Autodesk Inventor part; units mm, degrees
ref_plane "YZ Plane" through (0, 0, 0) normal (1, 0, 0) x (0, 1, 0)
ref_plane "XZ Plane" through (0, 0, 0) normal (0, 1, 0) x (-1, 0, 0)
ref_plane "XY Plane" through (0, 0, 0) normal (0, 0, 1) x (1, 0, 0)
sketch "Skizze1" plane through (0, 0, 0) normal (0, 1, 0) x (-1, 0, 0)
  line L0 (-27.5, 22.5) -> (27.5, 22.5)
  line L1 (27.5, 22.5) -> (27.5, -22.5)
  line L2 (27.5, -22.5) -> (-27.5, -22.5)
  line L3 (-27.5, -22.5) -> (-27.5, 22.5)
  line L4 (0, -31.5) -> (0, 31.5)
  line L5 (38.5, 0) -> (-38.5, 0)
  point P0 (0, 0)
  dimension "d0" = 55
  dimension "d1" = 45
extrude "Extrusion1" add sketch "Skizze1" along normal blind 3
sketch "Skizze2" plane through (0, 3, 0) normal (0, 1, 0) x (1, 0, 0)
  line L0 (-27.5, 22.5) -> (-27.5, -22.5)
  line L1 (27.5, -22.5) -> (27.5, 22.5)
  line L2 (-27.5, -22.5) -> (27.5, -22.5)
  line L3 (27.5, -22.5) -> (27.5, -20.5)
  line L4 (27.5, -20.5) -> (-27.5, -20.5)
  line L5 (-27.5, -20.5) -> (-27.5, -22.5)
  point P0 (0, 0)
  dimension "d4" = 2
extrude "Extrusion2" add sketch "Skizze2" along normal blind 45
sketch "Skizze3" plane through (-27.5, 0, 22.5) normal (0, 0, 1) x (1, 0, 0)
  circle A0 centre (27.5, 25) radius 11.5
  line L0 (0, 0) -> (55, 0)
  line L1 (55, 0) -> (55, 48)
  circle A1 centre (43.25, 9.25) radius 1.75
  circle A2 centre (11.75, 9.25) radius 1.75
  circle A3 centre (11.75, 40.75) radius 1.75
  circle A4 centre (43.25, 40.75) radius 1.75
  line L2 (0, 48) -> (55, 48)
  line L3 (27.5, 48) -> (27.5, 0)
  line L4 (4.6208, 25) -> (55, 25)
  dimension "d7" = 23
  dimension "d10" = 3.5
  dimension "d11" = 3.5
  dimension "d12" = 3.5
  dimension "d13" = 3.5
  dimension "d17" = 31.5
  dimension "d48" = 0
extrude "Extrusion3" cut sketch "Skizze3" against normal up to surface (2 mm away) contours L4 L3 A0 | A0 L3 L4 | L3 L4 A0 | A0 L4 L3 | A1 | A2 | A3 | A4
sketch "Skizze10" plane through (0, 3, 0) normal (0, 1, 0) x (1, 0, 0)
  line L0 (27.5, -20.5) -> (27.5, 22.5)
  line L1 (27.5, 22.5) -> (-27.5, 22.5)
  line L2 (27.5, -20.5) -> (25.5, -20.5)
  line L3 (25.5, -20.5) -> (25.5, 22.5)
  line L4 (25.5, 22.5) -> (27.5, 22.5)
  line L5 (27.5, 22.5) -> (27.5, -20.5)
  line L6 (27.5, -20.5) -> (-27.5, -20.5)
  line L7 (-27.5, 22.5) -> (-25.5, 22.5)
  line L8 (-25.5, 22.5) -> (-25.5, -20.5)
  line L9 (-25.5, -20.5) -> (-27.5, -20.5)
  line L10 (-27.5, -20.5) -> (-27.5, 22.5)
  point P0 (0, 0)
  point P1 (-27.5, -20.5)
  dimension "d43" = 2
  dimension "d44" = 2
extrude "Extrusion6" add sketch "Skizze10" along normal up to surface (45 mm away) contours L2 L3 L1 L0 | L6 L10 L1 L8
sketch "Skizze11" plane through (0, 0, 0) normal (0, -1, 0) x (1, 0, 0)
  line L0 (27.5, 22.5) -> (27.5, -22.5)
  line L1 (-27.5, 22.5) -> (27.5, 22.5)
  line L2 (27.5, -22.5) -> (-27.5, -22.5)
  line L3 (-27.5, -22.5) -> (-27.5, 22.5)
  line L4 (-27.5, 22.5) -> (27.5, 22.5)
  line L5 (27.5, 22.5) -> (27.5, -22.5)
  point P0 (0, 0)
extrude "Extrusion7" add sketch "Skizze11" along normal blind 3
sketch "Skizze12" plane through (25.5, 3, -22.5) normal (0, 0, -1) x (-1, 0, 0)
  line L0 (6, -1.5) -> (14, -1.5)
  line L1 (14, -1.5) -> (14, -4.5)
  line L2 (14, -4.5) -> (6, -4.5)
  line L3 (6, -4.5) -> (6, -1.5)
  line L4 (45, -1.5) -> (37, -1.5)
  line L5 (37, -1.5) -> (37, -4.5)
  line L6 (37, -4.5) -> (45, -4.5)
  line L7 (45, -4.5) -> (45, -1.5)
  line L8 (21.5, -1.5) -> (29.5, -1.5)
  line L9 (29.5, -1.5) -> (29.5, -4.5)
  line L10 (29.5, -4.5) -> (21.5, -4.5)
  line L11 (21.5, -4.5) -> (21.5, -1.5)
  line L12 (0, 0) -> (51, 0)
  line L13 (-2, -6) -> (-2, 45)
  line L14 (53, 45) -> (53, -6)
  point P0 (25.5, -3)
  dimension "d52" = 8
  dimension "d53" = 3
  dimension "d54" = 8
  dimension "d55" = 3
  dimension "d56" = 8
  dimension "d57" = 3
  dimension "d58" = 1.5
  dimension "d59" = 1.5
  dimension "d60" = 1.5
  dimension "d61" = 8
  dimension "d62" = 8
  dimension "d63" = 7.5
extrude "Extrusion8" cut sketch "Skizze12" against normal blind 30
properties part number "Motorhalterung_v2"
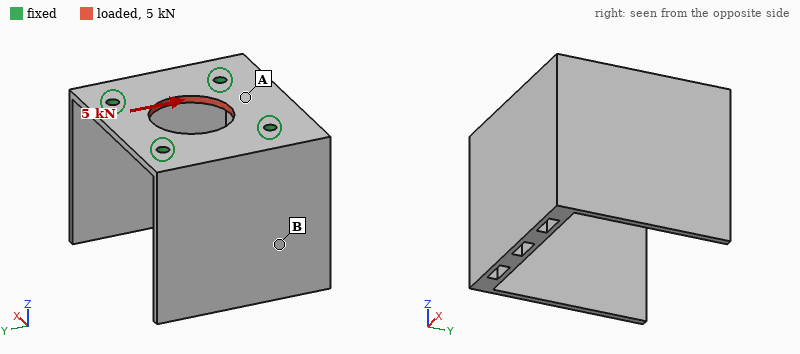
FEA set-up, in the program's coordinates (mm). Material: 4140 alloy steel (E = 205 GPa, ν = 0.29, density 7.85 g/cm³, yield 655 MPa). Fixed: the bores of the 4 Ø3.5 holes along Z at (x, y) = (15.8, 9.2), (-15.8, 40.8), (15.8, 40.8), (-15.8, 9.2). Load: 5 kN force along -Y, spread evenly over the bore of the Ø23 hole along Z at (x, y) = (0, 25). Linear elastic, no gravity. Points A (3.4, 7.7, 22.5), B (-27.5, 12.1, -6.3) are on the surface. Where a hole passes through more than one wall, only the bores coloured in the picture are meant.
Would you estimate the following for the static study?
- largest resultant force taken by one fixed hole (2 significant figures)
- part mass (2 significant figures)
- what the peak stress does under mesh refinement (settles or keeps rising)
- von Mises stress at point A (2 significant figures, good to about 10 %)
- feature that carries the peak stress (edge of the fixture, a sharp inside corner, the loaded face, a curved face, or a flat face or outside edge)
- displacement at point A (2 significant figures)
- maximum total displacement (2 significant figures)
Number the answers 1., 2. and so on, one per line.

1. 1.3 kN
2. 190 g
3. keeps rising
4. 25 MPa
5. edge of the fixture
6. 3.3 µm
7. 6.6 µm
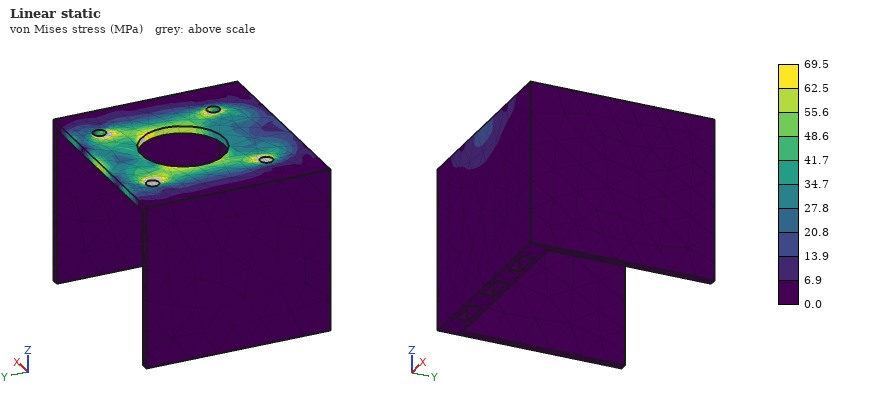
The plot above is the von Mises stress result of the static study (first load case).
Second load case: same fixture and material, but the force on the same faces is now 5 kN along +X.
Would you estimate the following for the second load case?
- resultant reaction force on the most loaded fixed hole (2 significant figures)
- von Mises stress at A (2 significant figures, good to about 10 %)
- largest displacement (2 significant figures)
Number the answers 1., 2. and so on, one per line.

1. 1.3 kN
2. 25 MPa
3. 4.8 µm
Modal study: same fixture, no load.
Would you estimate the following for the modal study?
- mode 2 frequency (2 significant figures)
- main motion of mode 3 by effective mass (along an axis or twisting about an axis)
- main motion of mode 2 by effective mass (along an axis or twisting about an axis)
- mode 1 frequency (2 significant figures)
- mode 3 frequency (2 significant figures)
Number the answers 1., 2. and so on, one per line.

1. 1400 Hz
2. along Y
3. along X
4. 1400 Hz
5. 2200 Hz
